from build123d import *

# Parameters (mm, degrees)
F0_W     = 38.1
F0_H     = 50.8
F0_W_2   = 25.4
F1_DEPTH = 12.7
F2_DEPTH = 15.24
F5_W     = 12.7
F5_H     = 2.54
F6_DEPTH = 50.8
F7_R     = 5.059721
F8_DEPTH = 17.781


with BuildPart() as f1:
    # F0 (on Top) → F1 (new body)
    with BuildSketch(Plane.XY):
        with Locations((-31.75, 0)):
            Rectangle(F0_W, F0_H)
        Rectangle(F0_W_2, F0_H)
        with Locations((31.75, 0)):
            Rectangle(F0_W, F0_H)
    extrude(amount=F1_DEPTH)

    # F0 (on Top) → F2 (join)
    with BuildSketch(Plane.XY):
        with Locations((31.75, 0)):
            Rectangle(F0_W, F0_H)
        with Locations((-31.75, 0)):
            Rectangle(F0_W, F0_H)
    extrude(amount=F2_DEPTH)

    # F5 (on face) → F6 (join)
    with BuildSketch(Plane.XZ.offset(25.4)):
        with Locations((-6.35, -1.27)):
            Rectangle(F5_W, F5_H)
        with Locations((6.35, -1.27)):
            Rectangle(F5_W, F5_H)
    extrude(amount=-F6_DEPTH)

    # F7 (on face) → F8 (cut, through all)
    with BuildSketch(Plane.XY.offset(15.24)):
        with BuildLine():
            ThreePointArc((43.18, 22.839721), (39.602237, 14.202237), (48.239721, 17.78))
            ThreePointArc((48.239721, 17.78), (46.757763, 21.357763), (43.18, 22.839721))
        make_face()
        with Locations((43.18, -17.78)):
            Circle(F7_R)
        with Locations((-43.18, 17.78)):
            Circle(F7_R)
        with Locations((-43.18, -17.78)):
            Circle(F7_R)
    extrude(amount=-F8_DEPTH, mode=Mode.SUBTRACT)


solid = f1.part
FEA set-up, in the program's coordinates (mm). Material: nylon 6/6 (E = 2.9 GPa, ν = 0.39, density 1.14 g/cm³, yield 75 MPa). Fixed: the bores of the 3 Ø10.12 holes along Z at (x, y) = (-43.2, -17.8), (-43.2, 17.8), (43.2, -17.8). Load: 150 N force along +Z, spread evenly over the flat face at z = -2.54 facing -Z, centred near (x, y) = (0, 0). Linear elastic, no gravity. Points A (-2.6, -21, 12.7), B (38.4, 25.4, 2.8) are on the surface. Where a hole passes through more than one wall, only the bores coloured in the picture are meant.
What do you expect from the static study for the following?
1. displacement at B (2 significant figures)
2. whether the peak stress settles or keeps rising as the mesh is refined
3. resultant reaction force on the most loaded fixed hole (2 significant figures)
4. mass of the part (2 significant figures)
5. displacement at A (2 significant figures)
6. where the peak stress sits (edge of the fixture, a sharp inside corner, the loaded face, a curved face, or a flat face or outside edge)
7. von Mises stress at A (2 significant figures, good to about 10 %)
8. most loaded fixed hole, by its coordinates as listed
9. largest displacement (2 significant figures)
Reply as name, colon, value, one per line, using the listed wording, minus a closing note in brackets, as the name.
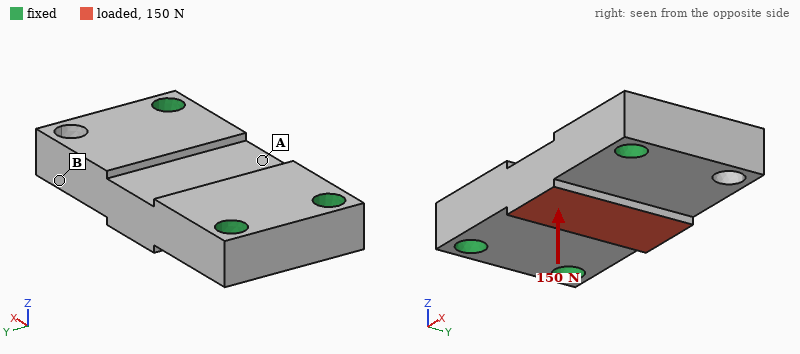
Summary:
displacement at B: 16 µm
whether the peak stress settles or keeps rising as the mesh is refined: keeps rising
resultant reaction force on the most loaded fixed hole: 73 N
mass of the part: 84 g
displacement at A: 13 µm
where the peak stress sits: edge of the fixture
von Mises stress at A: 0.49 MPa
most loaded fixed hole, by its coordinates as listed: (43.2, -17.8)
largest displacement: 26 µm
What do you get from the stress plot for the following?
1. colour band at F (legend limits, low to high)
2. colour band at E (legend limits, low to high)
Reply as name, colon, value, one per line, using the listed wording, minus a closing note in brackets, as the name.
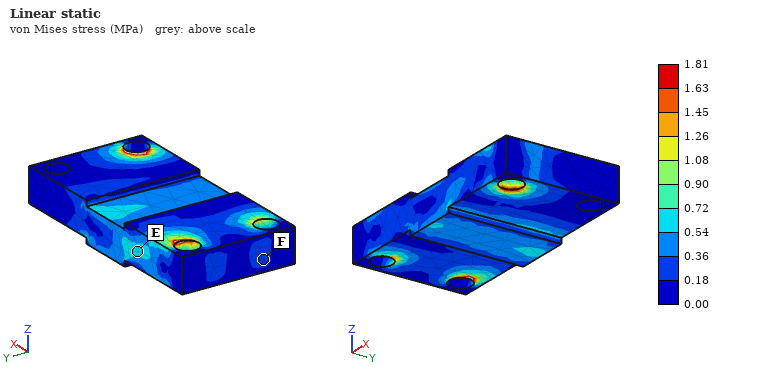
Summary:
colour band at F: 0.18 to 0.36 MPa
colour band at E: 0.54 to 0.72 MPa
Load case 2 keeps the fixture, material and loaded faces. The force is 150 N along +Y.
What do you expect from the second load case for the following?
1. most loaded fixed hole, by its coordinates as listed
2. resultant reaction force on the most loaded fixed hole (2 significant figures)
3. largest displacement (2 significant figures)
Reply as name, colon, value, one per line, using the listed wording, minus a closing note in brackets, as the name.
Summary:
most loaded fixed hole, by its coordinates as listed: (-43.2, -17.8)
resultant reaction force on the most loaded fixed hole: 85 N
largest displacement: 19 µm
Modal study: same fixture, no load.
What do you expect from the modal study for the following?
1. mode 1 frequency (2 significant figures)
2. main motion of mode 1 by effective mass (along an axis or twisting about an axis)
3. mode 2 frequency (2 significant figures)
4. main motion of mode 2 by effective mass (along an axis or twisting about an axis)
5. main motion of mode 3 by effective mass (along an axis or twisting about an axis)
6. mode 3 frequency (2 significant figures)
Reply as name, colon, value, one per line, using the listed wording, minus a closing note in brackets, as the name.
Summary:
mode 1 frequency: 2000 Hz
main motion of mode 1 by effective mass: along Z
mode 2 frequency: 3200 Hz
main motion of mode 2 by effective mass: along Z
main motion of mode 3 by effective mass: along Y
mode 3 frequency: 4100 Hz
